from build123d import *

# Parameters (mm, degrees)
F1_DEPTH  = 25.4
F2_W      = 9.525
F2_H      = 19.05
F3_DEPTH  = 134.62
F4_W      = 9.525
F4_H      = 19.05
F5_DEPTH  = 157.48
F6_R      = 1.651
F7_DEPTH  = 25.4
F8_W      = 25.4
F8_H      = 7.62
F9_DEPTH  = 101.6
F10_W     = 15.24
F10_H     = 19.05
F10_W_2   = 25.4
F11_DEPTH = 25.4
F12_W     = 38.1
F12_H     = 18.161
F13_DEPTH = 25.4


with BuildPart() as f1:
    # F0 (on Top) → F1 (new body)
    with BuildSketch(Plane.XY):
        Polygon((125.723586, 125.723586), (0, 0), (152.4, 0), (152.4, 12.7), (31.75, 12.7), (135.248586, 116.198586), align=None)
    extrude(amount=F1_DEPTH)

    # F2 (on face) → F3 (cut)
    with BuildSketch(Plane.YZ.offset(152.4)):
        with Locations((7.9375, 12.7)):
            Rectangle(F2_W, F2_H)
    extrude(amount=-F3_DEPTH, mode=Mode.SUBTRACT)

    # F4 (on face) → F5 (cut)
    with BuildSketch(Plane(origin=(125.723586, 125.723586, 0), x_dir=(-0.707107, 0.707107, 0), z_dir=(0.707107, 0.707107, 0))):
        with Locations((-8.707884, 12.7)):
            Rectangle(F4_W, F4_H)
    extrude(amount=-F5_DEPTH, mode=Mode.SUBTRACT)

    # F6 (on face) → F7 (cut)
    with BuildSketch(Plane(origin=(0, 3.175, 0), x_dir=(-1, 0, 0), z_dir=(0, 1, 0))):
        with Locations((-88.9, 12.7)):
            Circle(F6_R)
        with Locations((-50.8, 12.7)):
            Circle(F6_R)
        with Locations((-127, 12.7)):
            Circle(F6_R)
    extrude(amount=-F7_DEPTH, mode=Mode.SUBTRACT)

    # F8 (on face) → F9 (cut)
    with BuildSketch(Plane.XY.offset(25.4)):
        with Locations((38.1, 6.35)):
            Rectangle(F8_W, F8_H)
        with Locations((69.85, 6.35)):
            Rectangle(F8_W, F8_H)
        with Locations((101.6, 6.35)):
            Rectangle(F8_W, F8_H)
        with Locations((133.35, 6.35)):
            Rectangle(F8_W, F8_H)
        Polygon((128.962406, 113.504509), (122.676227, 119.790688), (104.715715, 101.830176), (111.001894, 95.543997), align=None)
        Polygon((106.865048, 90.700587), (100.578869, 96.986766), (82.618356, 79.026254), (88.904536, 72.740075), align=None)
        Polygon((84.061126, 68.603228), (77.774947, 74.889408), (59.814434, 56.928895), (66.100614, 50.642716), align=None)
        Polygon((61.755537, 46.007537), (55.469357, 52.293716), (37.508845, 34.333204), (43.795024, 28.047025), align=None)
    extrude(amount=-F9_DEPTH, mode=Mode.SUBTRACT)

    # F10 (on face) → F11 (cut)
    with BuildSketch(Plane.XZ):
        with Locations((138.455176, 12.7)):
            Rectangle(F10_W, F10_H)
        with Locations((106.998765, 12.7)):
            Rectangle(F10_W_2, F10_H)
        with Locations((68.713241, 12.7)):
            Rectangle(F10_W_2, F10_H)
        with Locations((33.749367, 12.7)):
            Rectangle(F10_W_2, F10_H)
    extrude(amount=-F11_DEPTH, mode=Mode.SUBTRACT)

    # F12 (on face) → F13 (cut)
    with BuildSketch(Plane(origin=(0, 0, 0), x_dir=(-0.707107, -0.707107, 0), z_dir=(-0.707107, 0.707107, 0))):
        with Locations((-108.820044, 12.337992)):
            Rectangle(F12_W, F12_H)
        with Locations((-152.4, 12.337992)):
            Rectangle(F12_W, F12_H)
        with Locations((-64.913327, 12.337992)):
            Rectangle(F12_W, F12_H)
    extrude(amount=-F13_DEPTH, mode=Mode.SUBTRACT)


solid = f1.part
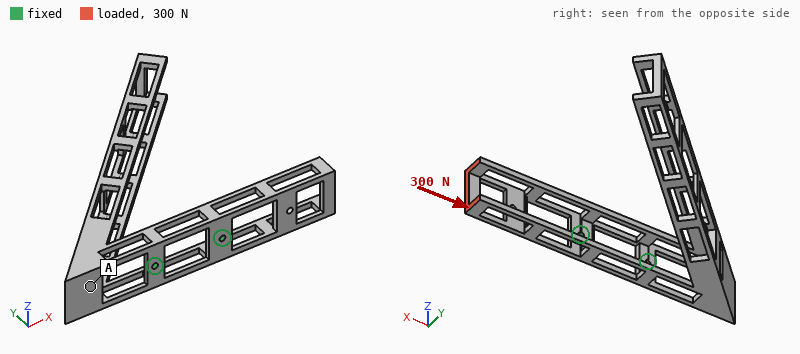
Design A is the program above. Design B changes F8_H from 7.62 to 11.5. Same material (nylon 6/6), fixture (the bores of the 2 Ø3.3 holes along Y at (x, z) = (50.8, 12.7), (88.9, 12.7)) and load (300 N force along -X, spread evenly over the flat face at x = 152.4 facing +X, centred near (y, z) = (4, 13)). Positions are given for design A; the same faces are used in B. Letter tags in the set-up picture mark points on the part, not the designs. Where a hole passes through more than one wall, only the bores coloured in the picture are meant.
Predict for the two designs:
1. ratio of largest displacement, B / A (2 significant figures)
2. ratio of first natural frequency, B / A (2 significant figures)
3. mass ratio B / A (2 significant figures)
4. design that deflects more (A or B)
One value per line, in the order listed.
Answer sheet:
3.7
0.38
0.85
B
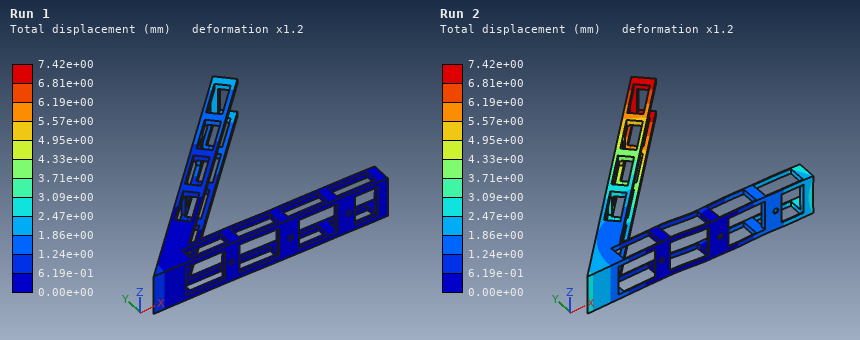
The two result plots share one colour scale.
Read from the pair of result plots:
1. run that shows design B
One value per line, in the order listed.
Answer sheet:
Run 2
